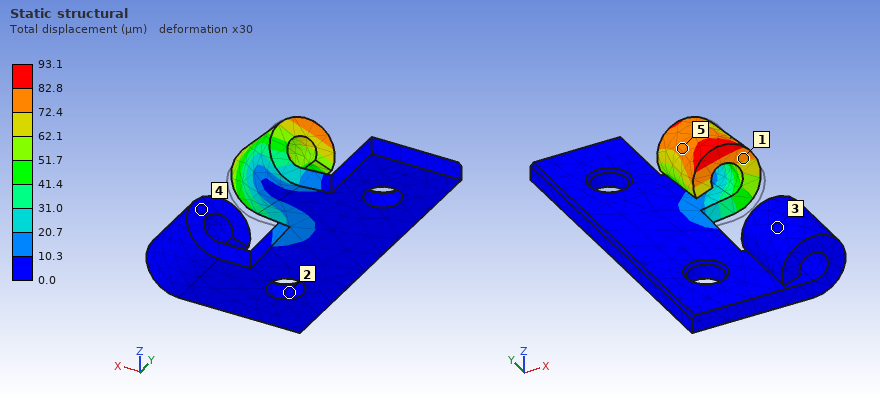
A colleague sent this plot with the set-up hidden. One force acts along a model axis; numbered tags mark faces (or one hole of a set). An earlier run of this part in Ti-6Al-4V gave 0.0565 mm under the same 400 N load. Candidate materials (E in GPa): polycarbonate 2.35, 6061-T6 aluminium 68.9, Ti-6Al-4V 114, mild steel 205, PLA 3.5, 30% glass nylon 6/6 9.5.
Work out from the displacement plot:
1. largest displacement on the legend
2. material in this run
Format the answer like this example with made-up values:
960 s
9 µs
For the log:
93.1 µm
6061-T6 aluminium
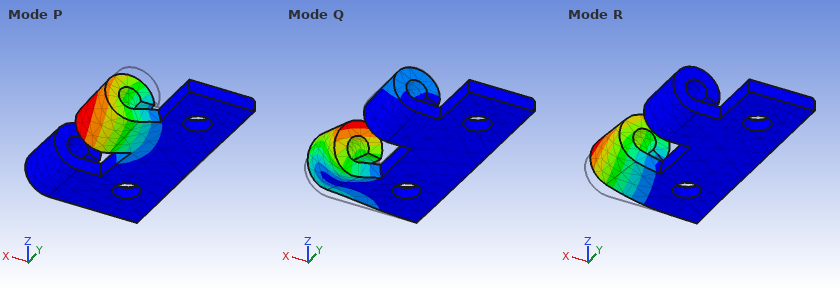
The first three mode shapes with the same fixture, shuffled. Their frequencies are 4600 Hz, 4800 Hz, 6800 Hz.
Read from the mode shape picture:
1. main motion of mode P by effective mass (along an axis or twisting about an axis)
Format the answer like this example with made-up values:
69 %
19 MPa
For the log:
along Z
